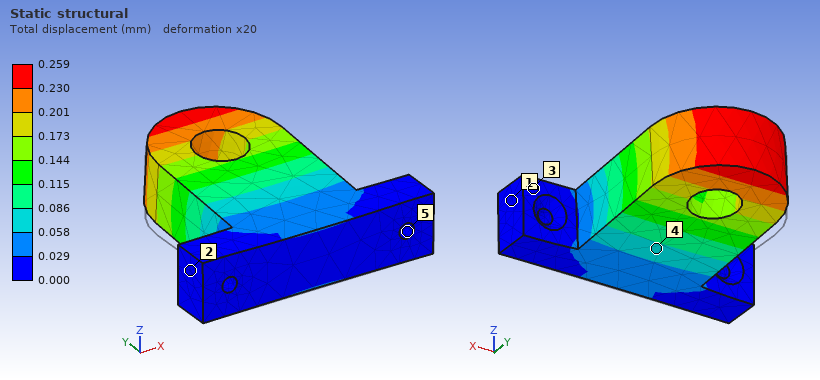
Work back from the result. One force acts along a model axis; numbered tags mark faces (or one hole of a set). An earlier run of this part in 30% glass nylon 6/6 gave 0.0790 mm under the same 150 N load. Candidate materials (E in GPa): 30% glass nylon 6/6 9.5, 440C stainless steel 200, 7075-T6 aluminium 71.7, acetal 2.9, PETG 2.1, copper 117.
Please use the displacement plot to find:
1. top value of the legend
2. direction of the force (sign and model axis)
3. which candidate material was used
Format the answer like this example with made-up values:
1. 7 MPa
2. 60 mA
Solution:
1. 0.259 mm
2. +Z
3. acetal
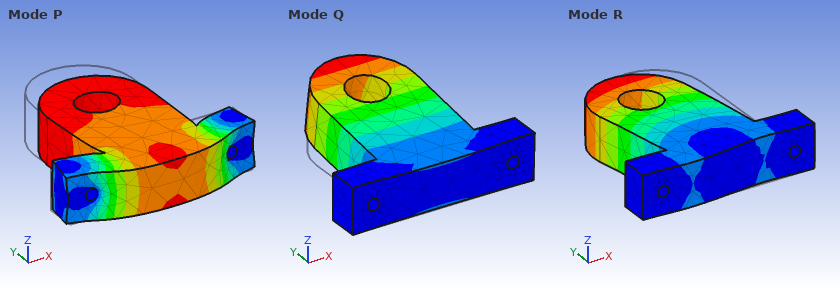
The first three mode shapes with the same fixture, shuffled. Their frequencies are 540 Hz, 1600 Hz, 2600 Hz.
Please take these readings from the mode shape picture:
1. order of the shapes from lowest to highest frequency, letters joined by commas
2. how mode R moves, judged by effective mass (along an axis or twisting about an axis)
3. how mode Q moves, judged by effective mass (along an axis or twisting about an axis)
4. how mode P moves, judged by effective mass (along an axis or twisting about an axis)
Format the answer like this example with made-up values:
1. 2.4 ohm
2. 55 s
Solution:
1. Q, R, P
2. along X
3. along Z
4. along Y
